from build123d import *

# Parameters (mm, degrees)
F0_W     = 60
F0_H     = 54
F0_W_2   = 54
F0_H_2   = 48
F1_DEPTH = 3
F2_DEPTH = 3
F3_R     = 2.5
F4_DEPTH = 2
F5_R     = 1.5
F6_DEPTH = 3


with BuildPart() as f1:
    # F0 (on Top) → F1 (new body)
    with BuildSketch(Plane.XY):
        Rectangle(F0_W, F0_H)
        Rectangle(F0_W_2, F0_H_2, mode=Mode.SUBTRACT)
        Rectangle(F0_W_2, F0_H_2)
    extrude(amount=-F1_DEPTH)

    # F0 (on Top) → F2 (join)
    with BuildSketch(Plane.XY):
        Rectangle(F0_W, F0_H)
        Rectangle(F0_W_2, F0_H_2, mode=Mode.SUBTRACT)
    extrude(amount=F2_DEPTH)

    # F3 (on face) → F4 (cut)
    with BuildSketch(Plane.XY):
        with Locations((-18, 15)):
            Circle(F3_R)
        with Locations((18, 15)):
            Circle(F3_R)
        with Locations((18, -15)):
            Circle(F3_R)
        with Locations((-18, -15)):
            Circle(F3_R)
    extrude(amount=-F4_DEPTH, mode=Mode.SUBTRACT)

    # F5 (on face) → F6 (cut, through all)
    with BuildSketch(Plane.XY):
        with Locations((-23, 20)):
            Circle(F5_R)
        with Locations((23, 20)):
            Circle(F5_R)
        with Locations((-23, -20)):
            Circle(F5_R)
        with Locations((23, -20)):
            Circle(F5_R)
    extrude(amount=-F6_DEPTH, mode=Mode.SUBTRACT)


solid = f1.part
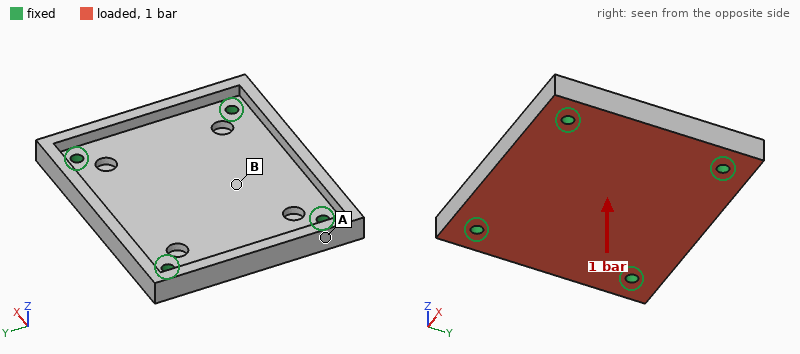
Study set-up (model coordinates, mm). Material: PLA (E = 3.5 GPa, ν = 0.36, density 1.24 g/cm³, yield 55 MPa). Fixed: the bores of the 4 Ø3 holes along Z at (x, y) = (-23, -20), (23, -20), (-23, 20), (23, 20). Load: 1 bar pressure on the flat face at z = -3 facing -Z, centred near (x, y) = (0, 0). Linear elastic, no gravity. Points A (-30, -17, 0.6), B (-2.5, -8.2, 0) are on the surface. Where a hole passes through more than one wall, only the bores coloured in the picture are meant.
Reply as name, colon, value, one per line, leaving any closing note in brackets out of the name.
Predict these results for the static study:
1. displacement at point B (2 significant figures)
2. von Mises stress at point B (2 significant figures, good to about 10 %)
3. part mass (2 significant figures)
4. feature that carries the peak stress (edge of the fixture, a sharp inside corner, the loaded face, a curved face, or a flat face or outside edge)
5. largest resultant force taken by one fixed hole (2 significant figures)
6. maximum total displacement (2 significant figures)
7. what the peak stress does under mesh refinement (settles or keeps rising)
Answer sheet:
displacement at point B: 0.22 mm
von Mises stress at point B: 5.6 MPa
part mass: 14 g
feature that carries the peak stress: edge of the fixture
largest resultant force taken by one fixed hole: 81 N
maximum total displacement: 0.25 mm
what the peak stress does under mesh refinement: keeps rising
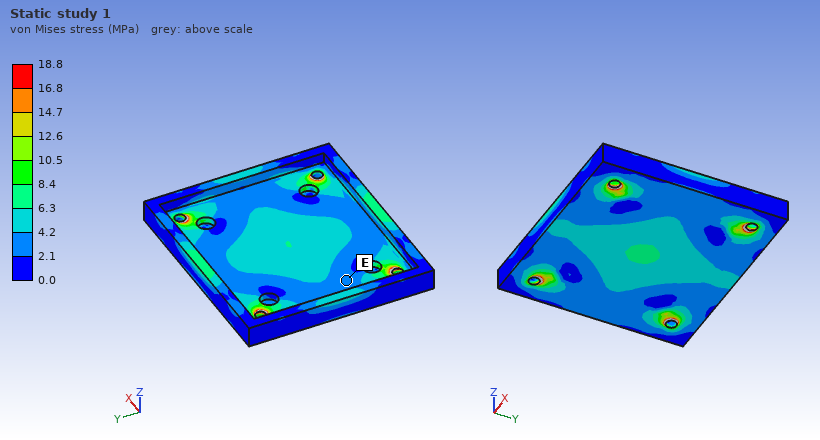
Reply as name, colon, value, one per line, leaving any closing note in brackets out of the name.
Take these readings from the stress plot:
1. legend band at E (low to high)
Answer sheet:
legend band at E: 2.1 to 4.2 MPa
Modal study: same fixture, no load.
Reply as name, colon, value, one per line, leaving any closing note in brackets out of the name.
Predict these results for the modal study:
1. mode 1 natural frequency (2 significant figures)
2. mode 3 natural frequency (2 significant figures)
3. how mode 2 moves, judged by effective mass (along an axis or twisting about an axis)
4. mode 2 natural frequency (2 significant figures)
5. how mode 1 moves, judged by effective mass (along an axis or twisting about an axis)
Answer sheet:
mode 1 natural frequency: 2000 Hz
mode 3 natural frequency: 3400 Hz
how mode 2 moves, judged by effective mass: twisting about X
mode 2 natural frequency: 3100 Hz
how mode 1 moves, judged by effective mass: along Z
